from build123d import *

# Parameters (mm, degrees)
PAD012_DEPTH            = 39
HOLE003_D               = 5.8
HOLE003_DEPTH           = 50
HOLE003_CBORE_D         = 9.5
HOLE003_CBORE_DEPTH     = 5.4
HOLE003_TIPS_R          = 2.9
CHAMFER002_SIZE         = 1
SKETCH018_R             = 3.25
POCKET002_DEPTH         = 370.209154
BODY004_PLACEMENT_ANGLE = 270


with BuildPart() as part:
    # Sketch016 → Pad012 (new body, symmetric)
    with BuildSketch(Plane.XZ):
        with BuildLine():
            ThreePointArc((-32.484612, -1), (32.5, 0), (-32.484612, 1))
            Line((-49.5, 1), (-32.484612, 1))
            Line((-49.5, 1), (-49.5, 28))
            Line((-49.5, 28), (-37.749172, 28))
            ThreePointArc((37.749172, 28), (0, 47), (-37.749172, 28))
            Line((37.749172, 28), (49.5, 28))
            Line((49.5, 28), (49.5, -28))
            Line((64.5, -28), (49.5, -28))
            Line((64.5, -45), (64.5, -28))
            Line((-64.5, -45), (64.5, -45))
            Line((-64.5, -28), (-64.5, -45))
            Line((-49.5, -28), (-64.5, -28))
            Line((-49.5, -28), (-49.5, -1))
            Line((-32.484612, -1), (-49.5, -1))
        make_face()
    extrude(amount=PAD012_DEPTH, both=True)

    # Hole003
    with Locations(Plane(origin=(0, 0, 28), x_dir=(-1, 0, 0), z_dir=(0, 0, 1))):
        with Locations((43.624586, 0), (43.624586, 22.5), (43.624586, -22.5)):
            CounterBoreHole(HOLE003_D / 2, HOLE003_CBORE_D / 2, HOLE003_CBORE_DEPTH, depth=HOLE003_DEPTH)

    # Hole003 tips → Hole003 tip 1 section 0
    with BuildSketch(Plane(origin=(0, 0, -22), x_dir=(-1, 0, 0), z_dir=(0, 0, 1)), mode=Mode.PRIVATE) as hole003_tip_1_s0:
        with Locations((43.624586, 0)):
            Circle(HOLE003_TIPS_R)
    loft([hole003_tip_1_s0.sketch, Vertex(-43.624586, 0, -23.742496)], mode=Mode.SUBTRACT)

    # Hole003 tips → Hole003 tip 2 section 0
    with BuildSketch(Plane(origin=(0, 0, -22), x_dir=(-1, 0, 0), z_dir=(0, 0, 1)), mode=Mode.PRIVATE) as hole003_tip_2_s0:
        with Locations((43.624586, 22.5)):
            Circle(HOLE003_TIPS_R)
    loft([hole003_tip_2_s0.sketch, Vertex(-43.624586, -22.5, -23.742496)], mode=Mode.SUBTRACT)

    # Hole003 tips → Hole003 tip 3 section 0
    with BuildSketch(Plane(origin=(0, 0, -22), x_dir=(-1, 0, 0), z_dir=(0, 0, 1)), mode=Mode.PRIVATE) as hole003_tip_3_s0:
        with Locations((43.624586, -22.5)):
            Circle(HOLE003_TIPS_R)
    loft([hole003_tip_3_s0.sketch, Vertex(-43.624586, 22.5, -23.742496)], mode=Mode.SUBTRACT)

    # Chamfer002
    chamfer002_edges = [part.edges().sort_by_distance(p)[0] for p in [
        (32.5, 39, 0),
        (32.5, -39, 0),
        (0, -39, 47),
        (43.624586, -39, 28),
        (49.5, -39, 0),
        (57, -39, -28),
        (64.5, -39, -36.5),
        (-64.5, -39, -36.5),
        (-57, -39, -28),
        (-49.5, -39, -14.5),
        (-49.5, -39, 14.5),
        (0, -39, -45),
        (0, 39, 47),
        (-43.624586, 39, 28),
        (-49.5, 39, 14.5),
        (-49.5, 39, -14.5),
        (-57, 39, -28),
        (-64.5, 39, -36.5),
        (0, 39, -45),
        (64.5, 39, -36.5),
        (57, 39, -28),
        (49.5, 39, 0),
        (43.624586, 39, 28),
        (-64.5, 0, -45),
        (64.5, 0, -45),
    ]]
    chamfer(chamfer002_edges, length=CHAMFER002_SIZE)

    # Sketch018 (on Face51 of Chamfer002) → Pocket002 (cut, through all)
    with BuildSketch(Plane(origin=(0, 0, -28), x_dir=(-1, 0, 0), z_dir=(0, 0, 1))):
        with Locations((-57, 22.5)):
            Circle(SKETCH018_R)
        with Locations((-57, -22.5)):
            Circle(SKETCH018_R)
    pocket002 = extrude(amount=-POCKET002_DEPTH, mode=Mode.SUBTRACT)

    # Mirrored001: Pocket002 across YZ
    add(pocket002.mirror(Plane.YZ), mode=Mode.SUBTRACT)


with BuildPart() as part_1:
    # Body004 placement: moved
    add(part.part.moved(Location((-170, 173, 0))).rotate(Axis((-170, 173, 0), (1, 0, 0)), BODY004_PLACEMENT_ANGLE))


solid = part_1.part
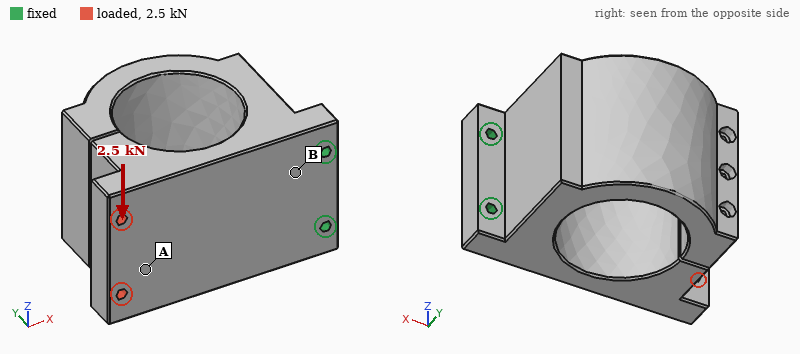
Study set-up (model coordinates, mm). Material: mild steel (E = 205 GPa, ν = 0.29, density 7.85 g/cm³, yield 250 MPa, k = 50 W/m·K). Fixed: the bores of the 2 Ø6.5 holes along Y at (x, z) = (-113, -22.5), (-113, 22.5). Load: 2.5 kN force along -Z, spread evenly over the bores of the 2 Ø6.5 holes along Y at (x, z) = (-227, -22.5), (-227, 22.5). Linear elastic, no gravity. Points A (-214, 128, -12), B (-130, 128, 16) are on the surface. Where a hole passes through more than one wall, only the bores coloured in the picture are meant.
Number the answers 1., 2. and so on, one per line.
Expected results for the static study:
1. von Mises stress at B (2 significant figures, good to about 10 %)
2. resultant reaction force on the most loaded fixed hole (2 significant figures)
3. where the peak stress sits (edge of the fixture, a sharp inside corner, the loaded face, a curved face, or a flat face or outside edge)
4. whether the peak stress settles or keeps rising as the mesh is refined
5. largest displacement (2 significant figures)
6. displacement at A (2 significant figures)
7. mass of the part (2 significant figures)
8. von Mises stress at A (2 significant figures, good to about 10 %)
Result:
1. 11 MPa
2. 5.9 kN
3. edge of the fixture
4. keeps rising
5. 18 µm
6. 13 µm
7. 3.2 kg
8. 5.0 MPa
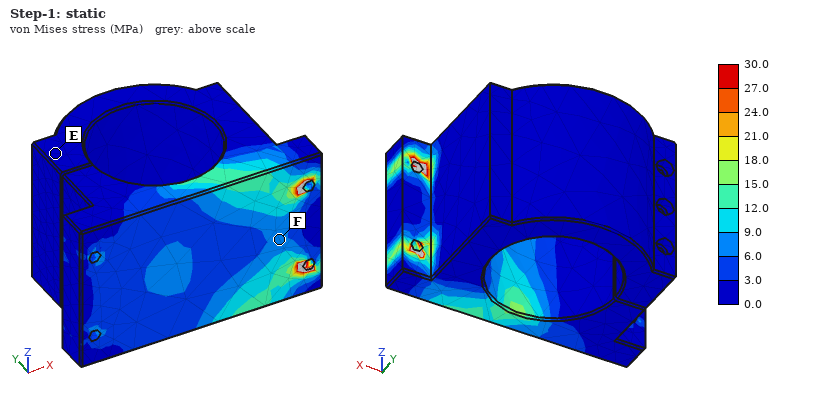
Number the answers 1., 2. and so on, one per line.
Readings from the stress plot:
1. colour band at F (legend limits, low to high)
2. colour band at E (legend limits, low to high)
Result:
1. 6.0 to 9.0 MPa
2. 0.0 to 3.0 MPa
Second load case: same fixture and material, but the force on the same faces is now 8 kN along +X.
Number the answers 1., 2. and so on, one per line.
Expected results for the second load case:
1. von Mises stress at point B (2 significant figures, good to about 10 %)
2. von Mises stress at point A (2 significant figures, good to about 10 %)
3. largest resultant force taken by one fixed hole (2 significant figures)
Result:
1. 8.8 MPa
2. 7.7 MPa
3. 4.0 kN
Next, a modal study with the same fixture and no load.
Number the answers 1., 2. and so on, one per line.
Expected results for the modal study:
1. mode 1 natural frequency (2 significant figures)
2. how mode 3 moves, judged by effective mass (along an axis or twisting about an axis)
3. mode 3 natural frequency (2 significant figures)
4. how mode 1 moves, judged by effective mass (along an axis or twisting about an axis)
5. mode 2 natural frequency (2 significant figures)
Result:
1. 550 Hz
2. along Z
3. 1100 Hz
4. along Y
5. 920 Hz
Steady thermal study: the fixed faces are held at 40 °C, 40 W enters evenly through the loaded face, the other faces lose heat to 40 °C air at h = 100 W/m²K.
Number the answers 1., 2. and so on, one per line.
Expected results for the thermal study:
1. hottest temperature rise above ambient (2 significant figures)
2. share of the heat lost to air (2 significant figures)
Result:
1. 29 K
2. 85 %
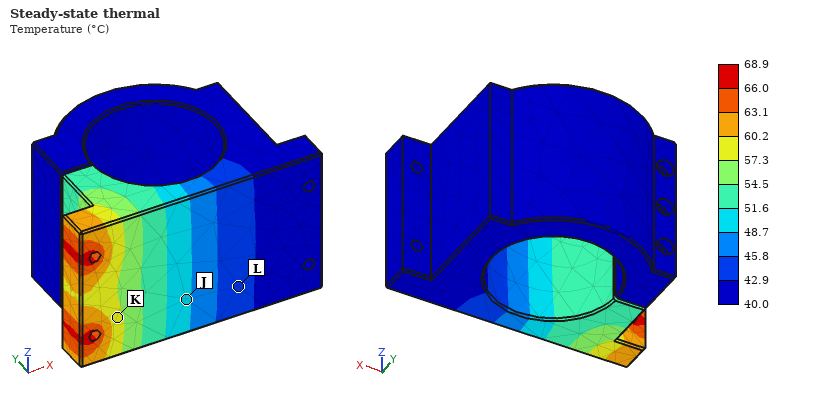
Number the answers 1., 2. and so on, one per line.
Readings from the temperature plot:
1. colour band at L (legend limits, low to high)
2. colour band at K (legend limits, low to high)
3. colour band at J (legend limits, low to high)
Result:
1. 42.9 to 45.8 °C
2. 57.3 to 60.2 °C
3. 48.7 to 51.6 °C
